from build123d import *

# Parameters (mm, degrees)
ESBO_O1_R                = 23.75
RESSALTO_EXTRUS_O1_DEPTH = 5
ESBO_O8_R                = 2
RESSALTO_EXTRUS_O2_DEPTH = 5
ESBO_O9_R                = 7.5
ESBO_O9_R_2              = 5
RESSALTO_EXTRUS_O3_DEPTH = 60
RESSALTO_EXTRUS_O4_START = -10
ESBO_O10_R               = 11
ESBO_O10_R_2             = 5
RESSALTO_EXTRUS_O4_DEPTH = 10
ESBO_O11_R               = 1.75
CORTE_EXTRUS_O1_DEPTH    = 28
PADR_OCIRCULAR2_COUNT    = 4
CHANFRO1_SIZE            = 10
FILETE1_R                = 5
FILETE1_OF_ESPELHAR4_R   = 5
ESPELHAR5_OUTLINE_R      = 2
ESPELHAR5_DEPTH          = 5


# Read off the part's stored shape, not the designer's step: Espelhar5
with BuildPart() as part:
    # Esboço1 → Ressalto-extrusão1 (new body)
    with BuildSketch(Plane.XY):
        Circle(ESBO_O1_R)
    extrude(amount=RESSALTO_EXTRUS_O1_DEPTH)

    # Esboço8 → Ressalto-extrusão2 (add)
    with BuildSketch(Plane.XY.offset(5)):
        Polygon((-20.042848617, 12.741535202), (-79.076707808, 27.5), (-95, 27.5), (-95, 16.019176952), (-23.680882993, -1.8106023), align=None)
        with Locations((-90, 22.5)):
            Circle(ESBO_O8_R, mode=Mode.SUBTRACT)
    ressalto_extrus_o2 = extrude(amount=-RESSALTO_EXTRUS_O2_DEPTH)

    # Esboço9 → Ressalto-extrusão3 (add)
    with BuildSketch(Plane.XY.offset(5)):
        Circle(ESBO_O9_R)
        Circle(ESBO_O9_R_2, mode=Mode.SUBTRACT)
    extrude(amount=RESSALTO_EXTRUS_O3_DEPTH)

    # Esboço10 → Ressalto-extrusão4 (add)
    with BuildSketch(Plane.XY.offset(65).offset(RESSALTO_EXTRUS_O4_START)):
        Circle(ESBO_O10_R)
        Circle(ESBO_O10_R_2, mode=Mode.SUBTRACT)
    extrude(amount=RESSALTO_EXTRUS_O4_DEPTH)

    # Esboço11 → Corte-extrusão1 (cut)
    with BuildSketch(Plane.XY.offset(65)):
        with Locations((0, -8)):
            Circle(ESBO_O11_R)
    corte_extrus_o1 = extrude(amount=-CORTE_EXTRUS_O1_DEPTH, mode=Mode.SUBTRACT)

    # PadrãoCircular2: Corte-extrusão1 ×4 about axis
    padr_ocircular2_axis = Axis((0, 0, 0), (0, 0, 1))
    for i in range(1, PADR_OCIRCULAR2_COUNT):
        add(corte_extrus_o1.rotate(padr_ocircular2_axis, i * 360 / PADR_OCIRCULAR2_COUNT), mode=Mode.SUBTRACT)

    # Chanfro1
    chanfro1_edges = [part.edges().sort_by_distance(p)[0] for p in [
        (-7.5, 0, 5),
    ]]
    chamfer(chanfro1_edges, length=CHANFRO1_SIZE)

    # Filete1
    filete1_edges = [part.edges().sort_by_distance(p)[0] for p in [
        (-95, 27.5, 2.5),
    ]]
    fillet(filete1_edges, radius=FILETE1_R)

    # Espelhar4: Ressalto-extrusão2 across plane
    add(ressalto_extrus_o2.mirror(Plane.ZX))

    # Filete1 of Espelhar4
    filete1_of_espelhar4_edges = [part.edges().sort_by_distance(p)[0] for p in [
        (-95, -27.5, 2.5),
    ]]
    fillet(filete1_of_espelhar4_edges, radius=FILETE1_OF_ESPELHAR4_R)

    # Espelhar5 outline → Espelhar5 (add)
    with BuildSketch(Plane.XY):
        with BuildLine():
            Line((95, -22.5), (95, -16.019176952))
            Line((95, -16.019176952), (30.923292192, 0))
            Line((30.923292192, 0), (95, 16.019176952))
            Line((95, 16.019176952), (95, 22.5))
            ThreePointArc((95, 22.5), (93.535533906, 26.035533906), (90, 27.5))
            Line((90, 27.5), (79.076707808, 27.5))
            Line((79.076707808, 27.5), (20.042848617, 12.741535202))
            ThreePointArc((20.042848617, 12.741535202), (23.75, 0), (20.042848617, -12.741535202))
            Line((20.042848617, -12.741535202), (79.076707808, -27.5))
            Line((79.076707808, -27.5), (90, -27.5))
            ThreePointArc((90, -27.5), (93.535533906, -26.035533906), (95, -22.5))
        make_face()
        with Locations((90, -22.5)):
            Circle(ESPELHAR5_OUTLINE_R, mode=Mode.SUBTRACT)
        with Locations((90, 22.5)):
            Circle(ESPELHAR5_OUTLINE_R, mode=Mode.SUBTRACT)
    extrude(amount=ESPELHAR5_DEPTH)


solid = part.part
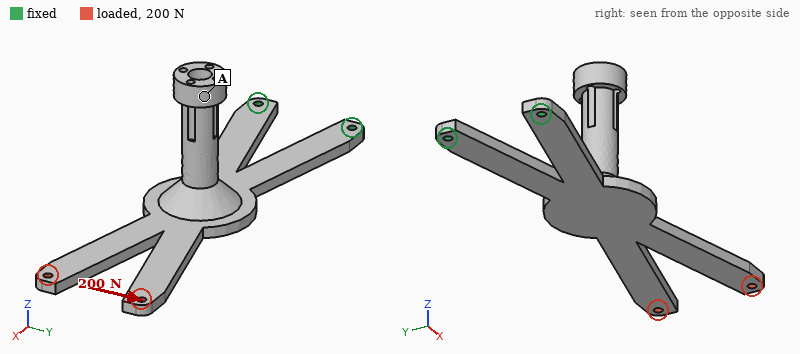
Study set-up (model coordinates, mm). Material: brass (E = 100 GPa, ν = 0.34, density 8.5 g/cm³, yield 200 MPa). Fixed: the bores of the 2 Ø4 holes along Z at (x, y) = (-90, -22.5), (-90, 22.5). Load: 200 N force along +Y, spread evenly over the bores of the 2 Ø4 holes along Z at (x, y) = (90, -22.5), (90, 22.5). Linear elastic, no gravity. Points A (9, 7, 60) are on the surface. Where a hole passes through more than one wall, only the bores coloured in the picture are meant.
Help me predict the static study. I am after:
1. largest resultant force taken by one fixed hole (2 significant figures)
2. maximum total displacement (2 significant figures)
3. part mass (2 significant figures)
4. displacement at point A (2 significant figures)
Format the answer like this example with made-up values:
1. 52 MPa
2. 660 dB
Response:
1. 870 N
2. 0.27 mm
3. 350 g
4. 0.042 mm
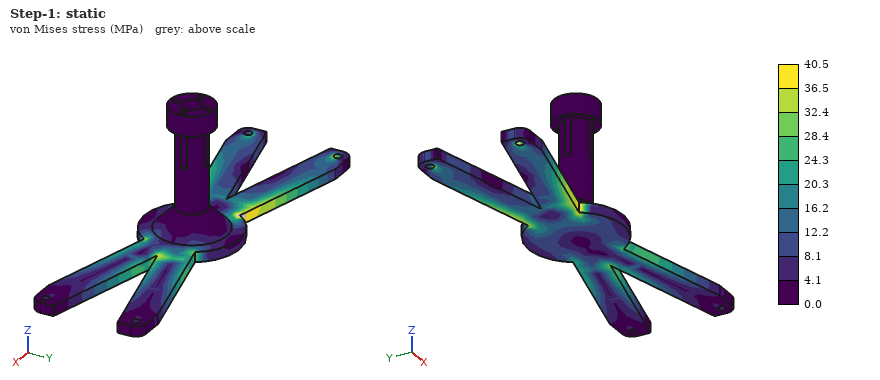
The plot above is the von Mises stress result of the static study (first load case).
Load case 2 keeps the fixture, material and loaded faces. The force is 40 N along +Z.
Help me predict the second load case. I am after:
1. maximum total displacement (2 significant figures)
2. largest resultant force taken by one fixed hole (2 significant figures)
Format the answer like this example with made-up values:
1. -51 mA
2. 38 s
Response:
1. 2.4 mm
2. 20 N
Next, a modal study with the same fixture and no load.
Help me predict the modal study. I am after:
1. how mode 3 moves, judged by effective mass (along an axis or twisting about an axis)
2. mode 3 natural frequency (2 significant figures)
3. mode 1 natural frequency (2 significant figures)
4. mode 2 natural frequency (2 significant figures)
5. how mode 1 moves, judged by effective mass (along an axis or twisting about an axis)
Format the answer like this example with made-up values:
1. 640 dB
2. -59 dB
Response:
1. along Z
2. 460 Hz
3. 74 Hz
4. 310 Hz
5. along Z
